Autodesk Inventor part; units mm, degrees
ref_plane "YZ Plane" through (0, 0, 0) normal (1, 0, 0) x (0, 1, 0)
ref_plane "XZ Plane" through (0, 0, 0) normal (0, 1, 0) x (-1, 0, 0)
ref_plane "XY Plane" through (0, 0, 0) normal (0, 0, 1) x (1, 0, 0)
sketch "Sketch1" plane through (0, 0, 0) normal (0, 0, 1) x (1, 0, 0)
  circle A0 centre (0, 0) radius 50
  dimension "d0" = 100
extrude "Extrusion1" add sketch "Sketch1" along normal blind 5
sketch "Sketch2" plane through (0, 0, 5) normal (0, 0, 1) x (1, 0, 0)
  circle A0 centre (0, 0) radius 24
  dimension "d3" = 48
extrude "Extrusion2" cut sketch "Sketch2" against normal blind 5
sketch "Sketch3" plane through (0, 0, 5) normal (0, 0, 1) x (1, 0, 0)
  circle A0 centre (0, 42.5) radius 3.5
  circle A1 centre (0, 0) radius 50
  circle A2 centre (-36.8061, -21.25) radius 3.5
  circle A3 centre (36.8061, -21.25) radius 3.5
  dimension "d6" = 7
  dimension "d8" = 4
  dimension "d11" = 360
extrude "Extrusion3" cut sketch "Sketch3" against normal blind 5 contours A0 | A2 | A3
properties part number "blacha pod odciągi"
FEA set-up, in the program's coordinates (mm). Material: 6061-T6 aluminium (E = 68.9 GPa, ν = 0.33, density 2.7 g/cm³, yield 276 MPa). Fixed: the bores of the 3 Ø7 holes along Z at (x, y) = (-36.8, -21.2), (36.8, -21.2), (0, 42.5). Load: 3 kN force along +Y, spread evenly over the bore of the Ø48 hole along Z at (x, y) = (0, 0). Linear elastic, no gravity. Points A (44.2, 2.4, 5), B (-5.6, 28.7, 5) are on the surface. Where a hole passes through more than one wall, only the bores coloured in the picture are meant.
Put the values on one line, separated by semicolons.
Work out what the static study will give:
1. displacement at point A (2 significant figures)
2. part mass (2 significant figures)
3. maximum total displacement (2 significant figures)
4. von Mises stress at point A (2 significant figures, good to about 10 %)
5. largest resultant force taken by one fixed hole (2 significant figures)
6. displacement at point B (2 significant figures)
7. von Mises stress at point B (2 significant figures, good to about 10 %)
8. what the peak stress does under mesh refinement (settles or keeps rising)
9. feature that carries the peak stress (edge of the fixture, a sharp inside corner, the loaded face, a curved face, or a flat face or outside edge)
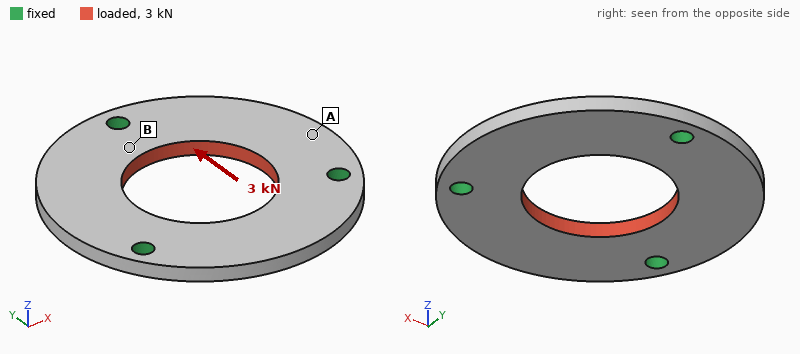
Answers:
2.0 µm; 80 g; 6.7 µm; 3.8 MPa; 1.1 kN; 1.6 µm; 7.8 MPa; keeps rising; edge of the fixture
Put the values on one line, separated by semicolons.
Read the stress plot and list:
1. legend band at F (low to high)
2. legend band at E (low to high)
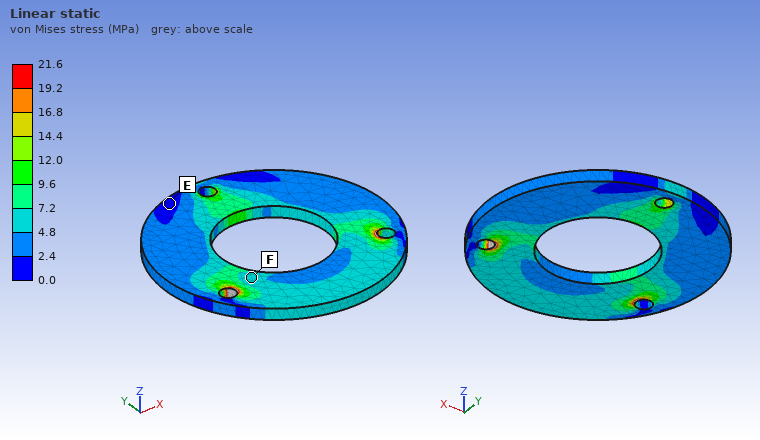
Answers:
4.8 to 7.2 MPa; 0.0 to 2.4 MPa
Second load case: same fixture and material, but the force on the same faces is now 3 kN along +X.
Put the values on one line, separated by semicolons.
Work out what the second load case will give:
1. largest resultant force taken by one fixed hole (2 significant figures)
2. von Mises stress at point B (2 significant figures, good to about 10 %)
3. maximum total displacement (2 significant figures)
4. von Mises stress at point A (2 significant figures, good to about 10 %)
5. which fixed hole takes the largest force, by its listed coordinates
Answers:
1.2 kN; 6.1 MPa; 6.0 µm; 4.5 MPa; (0, 42.5)
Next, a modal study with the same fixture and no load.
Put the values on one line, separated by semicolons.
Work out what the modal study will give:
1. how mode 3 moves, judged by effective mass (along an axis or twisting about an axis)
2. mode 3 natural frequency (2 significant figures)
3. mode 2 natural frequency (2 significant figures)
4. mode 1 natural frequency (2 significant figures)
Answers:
along Z; 3600 Hz; 3400 Hz; 3400 Hz
